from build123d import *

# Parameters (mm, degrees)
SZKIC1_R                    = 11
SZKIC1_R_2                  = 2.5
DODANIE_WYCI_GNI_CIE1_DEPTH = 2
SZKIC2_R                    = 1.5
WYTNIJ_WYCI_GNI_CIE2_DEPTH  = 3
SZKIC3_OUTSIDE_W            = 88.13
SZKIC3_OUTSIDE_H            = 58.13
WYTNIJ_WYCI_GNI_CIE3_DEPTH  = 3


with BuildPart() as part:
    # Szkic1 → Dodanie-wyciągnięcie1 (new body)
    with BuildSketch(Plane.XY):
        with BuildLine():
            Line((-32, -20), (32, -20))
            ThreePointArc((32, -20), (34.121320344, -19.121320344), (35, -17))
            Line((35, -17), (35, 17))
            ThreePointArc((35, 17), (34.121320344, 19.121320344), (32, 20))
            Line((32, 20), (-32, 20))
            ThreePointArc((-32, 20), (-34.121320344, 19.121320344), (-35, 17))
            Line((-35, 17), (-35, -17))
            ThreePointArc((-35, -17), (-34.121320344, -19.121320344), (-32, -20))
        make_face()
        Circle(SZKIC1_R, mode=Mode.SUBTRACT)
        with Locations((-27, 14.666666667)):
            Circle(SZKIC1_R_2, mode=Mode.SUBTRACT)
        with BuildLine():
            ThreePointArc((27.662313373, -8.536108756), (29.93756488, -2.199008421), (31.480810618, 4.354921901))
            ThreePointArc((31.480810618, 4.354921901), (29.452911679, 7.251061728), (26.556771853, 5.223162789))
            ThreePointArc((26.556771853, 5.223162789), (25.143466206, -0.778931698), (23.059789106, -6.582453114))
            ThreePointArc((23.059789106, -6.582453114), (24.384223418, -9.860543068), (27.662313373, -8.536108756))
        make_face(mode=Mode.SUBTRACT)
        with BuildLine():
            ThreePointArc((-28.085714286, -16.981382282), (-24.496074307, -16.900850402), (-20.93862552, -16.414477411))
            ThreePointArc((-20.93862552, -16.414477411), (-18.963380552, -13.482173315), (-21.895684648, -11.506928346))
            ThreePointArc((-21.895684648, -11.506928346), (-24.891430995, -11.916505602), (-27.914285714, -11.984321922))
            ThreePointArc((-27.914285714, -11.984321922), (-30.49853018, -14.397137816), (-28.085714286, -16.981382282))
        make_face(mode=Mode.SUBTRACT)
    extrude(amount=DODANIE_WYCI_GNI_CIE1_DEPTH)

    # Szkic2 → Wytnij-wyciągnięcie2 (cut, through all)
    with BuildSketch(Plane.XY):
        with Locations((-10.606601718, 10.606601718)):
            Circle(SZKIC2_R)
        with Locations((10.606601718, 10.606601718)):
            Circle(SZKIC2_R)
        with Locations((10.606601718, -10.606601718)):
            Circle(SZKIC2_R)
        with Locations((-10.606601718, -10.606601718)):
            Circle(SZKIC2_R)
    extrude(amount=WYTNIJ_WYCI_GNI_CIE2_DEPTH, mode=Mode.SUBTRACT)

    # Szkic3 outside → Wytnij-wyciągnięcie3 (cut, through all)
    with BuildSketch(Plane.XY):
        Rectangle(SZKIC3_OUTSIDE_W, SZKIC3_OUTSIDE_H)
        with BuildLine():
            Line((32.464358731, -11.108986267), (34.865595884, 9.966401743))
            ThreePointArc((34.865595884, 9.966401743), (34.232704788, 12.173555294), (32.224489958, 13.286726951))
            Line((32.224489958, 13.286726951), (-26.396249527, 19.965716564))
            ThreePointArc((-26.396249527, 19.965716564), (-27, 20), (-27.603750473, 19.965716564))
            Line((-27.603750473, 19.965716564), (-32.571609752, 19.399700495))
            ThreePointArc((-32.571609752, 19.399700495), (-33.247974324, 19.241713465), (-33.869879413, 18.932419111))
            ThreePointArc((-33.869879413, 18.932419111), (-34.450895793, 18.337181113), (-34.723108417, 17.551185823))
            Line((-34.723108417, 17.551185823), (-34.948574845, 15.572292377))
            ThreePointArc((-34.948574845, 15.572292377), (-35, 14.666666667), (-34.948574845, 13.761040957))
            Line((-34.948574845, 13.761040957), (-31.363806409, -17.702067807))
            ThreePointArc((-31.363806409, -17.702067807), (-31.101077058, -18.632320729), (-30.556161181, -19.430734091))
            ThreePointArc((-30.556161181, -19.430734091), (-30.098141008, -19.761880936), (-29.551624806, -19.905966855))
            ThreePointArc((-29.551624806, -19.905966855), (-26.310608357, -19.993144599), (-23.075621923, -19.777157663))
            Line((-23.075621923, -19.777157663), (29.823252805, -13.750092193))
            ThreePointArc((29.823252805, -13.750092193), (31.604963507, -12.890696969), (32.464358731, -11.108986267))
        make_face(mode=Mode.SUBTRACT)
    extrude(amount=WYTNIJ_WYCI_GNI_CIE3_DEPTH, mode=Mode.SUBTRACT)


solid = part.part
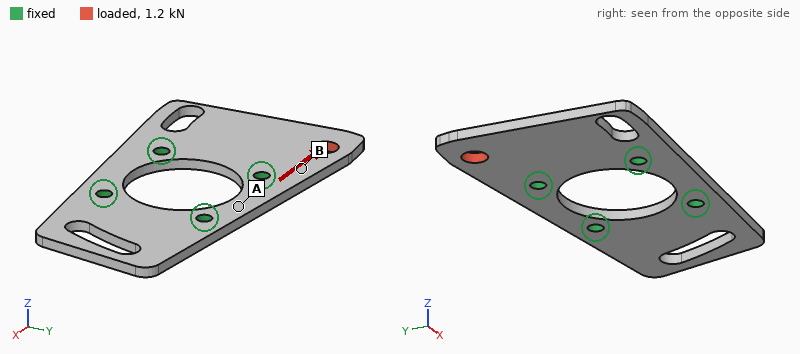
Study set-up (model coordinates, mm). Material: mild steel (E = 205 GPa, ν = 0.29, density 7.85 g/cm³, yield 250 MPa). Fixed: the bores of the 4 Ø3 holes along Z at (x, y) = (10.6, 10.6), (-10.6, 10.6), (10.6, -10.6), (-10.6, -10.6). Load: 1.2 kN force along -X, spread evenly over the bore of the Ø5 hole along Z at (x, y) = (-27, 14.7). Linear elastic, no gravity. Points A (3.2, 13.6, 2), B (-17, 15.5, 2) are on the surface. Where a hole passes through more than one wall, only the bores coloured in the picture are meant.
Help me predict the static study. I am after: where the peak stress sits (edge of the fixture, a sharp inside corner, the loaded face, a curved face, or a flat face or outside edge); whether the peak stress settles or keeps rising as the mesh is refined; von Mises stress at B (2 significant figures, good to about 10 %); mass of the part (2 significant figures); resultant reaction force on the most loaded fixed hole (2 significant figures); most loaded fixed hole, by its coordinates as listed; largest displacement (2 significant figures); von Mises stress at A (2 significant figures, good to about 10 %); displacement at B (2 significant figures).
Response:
edge of the fixture
keeps rising
53 MPa
27 g
1.2 kN
(-10.6, 10.6)
8.8 µm
14 MPa
3.2 µm
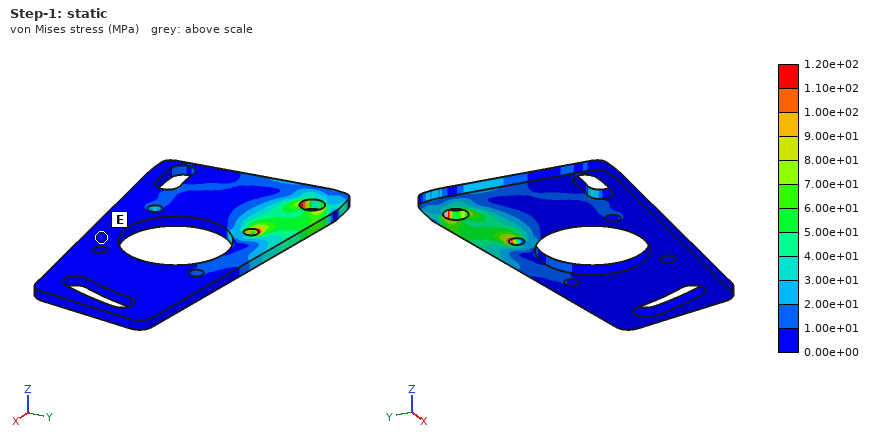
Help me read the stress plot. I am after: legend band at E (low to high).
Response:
0.00e+00 to 1.00e+01 MPa
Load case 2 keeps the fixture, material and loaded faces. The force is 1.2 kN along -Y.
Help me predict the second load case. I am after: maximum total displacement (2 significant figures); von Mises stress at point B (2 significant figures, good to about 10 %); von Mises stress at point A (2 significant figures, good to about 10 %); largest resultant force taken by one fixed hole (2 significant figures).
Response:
11 µm
21 MPa
14 MPa
950 N
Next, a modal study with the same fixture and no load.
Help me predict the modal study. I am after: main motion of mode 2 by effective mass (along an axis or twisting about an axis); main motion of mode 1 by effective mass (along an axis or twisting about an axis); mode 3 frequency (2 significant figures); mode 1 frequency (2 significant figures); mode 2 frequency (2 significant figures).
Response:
along Z
along Z
5600 Hz
3000 Hz
3400 Hz
